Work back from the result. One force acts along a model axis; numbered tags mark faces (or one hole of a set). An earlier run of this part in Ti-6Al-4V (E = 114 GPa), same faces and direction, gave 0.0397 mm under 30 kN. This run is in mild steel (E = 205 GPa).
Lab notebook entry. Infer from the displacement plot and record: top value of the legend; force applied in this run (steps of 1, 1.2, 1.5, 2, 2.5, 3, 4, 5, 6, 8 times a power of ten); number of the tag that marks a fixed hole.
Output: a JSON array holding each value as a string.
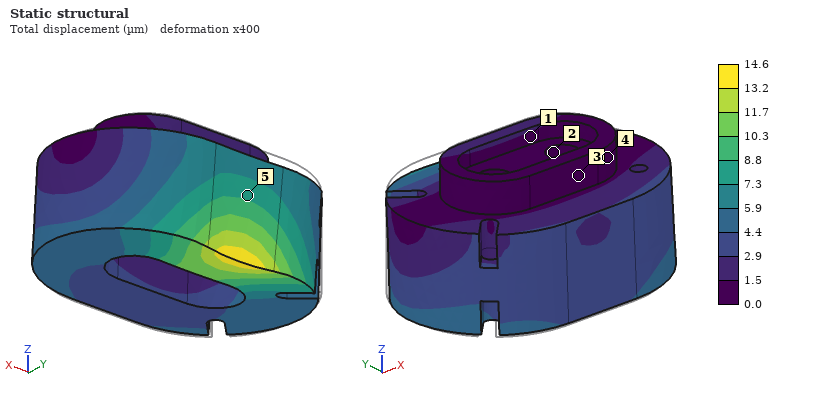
["14.6 µm", "20 kN", "2"]
